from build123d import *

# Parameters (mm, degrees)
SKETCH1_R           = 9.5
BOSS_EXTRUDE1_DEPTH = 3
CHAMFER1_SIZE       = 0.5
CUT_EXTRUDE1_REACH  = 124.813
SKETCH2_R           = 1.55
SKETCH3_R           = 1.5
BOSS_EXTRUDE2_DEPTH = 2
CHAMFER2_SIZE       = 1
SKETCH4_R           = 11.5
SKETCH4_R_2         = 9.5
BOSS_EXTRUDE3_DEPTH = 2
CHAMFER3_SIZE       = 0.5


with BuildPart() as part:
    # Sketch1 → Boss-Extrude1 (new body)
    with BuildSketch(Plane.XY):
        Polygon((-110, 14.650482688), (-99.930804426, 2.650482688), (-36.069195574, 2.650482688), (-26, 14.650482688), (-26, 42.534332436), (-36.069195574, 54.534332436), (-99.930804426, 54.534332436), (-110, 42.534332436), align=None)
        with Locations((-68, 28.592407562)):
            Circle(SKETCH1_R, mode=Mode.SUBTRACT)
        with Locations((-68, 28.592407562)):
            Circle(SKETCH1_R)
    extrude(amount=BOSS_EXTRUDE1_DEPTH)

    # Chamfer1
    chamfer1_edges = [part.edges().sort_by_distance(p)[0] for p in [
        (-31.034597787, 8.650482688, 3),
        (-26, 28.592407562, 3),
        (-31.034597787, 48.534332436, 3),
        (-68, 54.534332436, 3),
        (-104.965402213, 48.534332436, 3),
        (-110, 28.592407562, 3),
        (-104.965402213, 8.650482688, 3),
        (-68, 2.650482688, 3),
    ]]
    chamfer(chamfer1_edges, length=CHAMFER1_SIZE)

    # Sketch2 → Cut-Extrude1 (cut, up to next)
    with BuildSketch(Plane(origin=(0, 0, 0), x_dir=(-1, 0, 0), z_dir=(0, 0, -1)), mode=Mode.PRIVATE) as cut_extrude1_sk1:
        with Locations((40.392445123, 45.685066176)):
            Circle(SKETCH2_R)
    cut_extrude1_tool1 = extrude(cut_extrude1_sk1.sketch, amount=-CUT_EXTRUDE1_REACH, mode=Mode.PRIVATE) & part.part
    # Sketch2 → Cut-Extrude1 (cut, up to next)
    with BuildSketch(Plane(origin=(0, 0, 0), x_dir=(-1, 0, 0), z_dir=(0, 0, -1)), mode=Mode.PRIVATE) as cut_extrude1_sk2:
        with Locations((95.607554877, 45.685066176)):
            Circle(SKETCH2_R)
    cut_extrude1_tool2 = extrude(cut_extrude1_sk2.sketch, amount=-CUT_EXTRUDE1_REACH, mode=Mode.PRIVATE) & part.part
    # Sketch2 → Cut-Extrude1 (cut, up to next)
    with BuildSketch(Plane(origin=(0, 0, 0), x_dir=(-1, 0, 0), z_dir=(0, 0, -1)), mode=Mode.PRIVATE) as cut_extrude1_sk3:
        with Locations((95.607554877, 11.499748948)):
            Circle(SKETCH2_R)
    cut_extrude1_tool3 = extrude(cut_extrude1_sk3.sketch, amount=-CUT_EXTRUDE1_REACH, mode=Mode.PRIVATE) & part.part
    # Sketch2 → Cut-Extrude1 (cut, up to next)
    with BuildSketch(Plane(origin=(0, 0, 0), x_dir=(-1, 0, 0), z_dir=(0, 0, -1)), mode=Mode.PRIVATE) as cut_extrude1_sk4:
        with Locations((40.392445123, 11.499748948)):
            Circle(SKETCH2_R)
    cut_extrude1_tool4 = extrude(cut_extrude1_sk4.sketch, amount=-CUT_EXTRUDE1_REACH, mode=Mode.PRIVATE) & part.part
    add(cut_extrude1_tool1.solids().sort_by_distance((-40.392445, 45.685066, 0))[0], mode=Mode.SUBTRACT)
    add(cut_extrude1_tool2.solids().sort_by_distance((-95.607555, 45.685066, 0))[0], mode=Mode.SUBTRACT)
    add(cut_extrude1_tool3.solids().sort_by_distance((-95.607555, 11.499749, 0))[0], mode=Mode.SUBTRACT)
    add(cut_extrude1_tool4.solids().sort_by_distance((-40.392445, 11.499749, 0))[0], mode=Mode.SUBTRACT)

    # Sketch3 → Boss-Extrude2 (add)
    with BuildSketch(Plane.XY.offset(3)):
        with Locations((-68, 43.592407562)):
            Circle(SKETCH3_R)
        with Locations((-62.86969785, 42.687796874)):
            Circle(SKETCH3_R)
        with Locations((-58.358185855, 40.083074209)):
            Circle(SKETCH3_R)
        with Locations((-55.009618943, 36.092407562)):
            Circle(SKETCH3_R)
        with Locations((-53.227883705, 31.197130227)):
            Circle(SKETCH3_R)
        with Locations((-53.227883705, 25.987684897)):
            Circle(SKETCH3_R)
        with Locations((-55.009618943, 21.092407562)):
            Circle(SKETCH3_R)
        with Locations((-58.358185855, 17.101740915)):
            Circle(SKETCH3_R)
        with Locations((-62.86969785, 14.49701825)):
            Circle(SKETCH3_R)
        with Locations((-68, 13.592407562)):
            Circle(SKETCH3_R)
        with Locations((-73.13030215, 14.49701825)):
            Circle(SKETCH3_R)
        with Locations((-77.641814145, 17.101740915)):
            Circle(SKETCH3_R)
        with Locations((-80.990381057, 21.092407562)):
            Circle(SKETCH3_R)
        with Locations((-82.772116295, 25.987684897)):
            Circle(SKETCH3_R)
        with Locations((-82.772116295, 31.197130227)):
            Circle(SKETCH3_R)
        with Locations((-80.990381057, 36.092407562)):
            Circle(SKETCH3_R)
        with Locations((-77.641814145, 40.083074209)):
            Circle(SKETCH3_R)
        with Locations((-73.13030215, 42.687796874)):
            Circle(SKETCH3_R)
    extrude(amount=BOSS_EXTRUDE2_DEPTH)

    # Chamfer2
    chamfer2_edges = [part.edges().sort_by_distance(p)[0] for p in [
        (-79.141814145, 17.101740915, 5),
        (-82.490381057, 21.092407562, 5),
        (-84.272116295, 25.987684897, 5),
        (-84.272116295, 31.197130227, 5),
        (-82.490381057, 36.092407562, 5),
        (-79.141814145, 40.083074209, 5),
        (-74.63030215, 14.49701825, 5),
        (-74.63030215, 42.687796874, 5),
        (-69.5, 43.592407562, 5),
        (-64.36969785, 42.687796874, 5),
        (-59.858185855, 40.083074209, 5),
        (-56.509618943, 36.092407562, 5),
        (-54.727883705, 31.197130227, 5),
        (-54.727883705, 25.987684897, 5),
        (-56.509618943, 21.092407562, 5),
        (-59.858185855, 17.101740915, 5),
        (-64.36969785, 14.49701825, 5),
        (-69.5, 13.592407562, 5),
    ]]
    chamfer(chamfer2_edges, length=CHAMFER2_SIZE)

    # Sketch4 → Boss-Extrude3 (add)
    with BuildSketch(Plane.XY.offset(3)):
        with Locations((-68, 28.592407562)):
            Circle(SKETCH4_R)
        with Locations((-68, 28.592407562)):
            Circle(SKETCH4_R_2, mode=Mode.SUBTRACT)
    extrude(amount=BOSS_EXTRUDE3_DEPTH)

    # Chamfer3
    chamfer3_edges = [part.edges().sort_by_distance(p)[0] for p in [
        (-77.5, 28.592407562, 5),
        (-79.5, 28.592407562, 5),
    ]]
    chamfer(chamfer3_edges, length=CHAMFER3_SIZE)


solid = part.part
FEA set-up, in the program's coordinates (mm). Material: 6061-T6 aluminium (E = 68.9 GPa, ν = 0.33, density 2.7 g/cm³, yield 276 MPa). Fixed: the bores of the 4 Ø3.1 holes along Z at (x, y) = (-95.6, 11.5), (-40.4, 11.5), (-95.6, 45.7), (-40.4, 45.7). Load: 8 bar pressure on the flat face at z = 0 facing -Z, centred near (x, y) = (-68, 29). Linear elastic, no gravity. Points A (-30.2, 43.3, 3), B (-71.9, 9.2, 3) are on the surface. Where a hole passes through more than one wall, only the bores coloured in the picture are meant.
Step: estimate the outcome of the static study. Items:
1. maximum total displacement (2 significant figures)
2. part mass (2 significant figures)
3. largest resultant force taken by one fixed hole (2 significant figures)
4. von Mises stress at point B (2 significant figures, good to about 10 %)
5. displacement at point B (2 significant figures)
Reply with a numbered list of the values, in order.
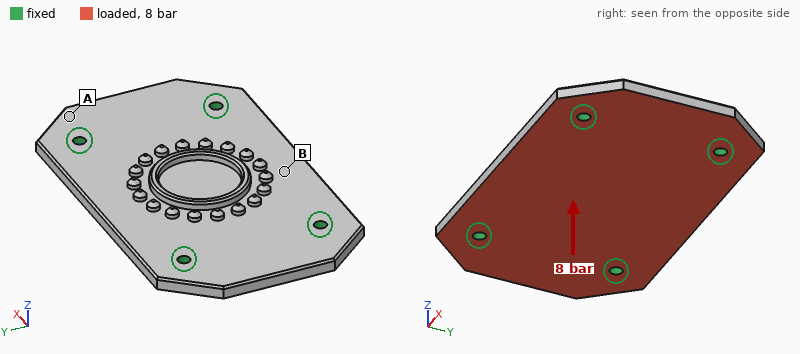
1. 0.14 mm
2. 34 g
3. 820 N
4. 61 MPa
5. 0.13 mm
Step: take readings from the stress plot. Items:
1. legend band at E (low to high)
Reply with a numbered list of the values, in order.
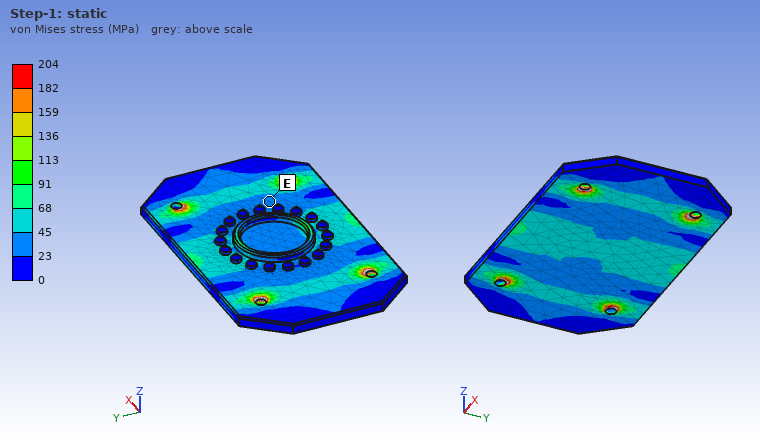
1. 23 to 45 MPa
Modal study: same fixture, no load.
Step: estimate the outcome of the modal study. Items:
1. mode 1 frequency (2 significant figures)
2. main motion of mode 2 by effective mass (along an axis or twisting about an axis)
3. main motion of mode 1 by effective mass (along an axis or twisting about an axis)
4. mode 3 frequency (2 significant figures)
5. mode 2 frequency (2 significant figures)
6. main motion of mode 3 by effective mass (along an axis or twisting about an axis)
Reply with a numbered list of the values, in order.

1. 4500 Hz
2. twisting about X
3. along Z
4. 8700 Hz
5. 5900 Hz
6. along Z
